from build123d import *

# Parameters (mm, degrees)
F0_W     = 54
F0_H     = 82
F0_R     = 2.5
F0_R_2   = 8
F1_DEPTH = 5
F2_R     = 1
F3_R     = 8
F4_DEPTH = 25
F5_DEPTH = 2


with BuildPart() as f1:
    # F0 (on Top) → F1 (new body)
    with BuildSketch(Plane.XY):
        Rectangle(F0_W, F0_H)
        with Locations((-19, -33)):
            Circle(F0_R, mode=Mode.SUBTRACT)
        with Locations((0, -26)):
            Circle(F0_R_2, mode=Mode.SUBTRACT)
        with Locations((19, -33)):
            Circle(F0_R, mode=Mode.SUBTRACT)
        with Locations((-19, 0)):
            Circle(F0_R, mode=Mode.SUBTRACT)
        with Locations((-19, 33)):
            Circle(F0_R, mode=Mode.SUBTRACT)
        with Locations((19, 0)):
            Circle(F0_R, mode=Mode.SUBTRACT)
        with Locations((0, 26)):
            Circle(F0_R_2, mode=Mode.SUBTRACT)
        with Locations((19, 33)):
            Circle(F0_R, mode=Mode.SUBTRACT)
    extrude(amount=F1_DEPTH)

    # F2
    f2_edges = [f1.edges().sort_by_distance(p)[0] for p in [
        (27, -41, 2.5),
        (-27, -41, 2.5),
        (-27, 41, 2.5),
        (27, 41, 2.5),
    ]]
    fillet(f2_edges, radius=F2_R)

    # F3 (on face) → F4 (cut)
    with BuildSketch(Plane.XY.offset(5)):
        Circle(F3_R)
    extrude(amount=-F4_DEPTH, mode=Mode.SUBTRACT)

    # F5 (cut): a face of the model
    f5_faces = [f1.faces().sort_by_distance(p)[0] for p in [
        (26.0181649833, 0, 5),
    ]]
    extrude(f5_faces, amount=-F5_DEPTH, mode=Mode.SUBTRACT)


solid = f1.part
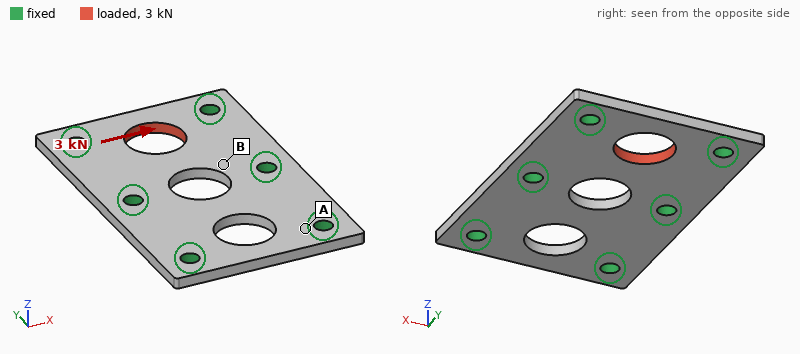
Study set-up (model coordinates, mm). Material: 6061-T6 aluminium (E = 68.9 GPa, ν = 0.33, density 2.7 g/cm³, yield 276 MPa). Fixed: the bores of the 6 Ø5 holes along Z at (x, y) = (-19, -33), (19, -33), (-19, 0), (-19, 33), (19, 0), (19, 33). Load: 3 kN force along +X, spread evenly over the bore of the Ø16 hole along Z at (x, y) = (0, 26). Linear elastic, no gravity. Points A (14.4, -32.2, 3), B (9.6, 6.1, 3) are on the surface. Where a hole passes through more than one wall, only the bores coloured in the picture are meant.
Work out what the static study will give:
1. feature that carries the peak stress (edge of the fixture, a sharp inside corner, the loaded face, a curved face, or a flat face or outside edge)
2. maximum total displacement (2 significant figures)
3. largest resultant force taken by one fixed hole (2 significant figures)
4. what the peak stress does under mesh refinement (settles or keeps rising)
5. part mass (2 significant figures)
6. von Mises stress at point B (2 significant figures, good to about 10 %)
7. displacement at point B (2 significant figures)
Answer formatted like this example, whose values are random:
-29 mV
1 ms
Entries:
edge of the fixture
6.6 µm
1.1 kN
keeps rising
30 g
12 MPa
2.1 µm
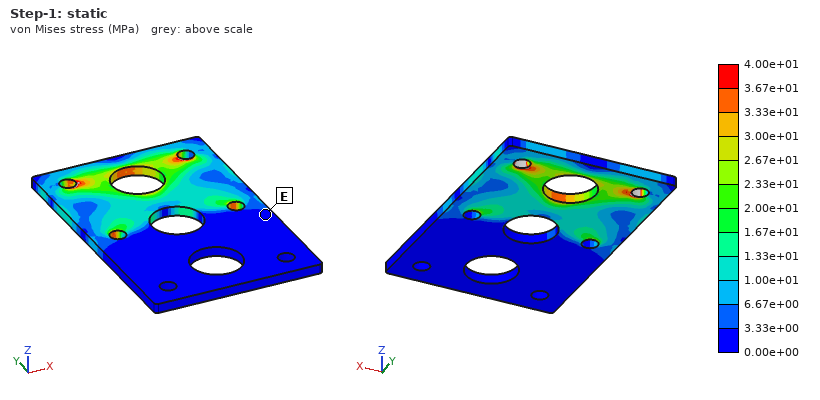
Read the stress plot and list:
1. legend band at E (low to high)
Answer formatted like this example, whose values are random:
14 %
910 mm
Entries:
0.00e+00 to 3.33e+00 MPa
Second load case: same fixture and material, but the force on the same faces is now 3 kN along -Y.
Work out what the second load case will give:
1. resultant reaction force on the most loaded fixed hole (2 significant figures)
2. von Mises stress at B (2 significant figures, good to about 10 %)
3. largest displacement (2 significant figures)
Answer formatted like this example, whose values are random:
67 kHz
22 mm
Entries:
880 N
16 MPa
16 µm
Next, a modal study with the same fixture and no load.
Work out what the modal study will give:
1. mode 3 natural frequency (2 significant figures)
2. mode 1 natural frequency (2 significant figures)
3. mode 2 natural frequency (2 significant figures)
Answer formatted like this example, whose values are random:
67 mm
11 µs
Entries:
13 kHz
10 kHz
10 kHz
